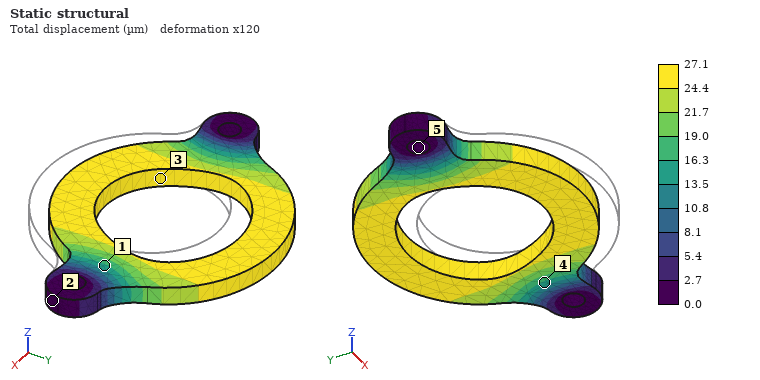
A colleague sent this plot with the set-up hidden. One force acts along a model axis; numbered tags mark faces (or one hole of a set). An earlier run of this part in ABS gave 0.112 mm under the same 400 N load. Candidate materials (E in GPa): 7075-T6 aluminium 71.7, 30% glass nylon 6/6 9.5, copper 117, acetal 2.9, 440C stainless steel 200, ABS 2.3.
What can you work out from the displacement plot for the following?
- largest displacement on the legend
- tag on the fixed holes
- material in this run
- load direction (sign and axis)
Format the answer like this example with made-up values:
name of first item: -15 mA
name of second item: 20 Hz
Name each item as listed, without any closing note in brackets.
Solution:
largest displacement on the legend: 27.1 µm
tag on the fixed holes: 5
material in this run: 30% glass nylon 6/6
load direction: +Y
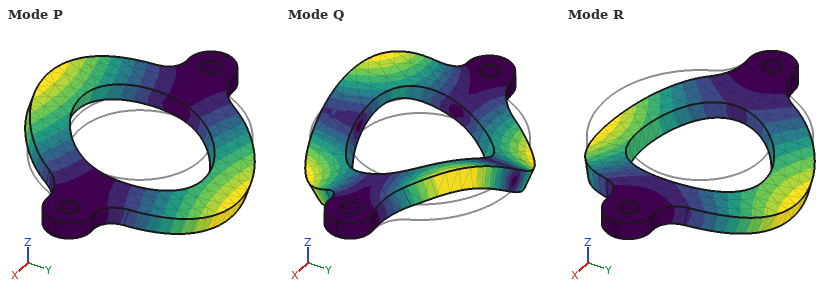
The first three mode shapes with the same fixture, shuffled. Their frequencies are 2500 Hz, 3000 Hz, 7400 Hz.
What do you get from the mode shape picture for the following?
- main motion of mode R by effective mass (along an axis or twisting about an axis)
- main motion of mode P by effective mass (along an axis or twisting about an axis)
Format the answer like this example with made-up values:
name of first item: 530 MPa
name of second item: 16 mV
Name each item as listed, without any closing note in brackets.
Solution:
main motion of mode R by effective mass: along Z
main motion of mode P by effective mass: twisting about X
